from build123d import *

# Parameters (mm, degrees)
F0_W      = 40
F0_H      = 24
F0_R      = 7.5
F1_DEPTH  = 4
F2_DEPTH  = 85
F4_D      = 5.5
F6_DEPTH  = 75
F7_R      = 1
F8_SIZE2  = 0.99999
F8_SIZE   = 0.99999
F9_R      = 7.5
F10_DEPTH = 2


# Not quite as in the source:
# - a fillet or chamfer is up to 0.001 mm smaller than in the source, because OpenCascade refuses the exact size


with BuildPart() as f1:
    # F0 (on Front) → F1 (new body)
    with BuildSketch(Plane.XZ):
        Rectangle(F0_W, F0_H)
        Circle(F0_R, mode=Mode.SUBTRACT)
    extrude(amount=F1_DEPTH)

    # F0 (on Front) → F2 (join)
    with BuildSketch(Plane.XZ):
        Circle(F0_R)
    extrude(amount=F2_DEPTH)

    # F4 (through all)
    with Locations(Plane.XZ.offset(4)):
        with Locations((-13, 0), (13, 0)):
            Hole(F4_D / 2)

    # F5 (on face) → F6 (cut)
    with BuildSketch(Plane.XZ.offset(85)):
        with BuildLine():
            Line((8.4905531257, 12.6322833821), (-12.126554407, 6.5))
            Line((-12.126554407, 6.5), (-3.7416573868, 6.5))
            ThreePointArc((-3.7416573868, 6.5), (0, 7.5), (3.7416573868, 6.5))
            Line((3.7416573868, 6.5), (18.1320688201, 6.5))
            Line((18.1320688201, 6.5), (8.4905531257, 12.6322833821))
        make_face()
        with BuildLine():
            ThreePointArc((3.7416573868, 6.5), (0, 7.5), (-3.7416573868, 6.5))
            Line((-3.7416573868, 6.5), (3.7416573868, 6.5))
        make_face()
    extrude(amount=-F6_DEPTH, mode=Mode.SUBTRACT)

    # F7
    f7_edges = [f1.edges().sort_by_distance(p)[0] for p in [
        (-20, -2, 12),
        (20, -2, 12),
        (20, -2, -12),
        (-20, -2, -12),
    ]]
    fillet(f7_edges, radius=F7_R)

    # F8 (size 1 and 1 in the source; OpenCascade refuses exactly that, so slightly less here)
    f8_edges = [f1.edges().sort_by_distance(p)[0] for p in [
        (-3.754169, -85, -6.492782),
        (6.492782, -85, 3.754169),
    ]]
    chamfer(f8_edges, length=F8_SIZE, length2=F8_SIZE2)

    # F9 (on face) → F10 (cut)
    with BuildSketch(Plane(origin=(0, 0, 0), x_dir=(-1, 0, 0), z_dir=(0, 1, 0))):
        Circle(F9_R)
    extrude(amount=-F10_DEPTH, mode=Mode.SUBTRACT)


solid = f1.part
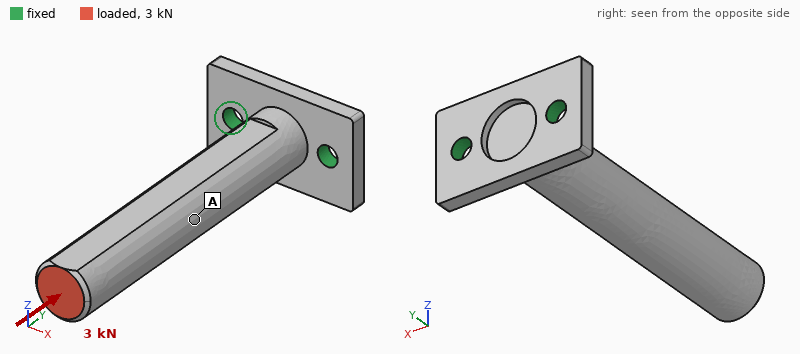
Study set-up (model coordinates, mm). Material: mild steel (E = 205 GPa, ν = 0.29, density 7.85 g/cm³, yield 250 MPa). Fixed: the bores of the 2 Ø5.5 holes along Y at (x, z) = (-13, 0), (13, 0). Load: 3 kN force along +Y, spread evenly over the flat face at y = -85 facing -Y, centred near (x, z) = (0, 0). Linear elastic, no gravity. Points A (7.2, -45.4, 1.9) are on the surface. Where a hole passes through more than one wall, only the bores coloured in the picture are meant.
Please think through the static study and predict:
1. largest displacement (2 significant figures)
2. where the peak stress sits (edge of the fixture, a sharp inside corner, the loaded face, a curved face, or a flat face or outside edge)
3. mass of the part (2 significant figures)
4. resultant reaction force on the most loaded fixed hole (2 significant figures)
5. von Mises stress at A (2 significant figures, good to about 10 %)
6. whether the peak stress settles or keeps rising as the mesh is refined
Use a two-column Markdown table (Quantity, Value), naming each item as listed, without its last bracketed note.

| Quantity | Value |
|---|---|
| largest displacement | 13 µm |
| where the peak stress sits | edge of the fixture |
| mass of the part | 140 g |
| resultant reaction force on the most loaded fixed hole | 1.7 kN |
| von Mises stress at A | 18 MPa |
| whether the peak stress settles or keeps rising as the mesh is refined | keeps rising |
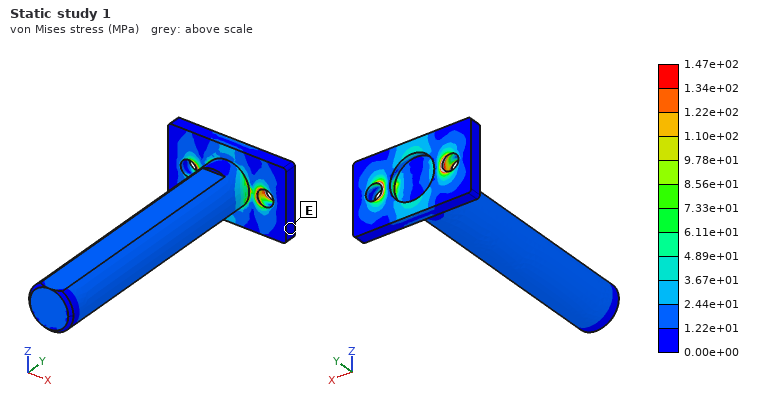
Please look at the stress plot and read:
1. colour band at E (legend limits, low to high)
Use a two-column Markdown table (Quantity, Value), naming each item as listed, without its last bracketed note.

| Quantity | Value |
|---|---|
| colour band at E | 0.00e+00 to 1.22e+01 MPa |
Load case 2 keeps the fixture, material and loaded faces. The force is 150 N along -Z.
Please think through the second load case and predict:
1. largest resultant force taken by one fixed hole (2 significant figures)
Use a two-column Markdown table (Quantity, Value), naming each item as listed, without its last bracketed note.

| Quantity | Value |
|---|---|
| largest resultant force taken by one fixed hole | 75 N |
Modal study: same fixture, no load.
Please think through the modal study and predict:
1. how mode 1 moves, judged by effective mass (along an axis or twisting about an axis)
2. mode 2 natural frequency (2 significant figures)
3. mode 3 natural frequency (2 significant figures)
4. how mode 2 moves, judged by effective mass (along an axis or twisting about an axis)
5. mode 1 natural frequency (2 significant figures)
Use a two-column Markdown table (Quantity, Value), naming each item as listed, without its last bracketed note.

| Quantity | Value |
|---|---|
| how mode 1 moves, judged by effective mass | along Z |
| mode 2 natural frequency | 1300 Hz |
| mode 3 natural frequency | 6700 Hz |
| how mode 2 moves, judged by effective mass | along X |
| mode 1 natural frequency | 840 Hz |
